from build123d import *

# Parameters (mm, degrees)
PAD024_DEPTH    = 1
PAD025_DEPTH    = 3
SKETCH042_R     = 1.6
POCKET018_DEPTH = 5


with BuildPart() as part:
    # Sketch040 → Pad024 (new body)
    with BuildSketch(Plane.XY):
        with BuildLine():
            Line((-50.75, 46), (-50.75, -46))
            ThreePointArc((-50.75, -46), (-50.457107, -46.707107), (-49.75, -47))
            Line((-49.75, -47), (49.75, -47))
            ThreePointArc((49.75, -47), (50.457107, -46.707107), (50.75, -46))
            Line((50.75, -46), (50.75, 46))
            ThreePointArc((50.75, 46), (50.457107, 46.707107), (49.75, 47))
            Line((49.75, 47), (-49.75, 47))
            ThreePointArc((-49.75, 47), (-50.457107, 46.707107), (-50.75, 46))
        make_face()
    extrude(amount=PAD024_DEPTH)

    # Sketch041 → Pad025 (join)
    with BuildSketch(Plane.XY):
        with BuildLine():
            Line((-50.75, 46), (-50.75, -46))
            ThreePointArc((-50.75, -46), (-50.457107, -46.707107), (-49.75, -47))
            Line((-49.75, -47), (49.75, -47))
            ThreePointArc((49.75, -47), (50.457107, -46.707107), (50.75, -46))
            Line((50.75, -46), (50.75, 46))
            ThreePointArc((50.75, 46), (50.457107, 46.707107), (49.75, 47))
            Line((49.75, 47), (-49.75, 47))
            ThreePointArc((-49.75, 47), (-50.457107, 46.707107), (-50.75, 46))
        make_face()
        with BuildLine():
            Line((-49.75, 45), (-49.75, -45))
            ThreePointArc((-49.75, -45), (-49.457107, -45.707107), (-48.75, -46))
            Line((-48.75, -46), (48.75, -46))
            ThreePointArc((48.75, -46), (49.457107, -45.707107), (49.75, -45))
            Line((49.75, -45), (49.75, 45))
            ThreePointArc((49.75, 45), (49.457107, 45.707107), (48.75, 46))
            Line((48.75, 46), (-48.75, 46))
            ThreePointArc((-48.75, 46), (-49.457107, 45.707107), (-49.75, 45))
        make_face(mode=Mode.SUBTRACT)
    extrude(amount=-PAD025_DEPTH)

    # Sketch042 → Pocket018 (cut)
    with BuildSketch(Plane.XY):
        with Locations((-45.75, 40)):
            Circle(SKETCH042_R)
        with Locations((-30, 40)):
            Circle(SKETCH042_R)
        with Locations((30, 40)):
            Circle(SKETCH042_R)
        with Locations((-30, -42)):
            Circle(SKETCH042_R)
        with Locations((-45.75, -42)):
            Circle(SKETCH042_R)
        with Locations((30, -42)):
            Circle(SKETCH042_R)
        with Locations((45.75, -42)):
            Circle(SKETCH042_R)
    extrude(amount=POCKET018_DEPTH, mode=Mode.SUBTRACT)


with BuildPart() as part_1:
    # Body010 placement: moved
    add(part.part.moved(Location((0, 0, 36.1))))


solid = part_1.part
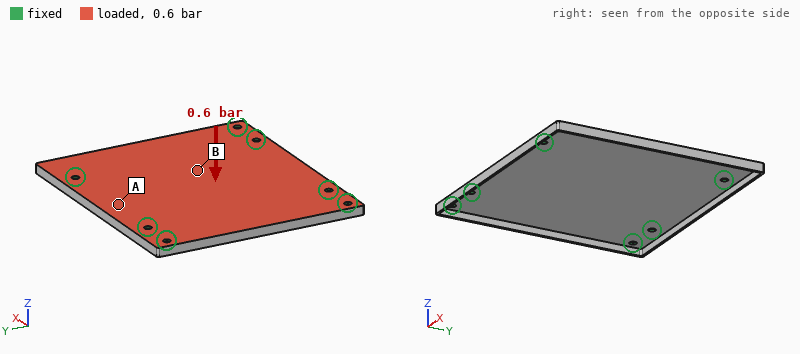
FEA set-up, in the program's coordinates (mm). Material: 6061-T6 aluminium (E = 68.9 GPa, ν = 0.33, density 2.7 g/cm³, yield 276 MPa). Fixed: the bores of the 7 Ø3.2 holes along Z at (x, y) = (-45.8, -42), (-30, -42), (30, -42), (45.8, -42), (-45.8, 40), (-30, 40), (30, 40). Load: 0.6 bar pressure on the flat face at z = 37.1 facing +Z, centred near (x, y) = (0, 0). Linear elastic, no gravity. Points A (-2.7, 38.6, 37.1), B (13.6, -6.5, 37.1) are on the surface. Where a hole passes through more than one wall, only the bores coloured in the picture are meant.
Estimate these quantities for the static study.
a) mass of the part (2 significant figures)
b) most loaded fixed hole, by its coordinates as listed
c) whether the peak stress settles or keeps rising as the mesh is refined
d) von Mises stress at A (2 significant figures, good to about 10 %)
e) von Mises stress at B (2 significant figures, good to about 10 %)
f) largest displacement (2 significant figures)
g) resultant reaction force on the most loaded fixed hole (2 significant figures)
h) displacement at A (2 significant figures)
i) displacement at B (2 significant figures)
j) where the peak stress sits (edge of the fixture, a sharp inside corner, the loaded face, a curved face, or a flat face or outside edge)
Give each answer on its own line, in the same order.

29 g
(30, 40)
keeps rising
39 MPa
91 MPa
1.6 mm
160 N
0.33 mm
1.4 mm
edge of the fixture
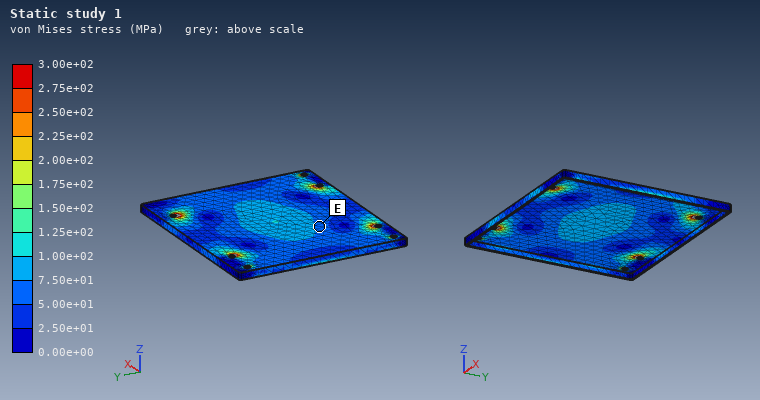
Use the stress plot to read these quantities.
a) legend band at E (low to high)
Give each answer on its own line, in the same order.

5.00e+01 to 7.50e+01 MPa
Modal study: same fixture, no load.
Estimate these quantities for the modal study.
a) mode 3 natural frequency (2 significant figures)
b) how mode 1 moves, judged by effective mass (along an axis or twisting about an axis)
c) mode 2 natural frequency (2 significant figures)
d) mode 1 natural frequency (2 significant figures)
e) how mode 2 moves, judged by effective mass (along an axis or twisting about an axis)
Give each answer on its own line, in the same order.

1600 Hz
along Z
1200 Hz
750 Hz
twisting about Y
